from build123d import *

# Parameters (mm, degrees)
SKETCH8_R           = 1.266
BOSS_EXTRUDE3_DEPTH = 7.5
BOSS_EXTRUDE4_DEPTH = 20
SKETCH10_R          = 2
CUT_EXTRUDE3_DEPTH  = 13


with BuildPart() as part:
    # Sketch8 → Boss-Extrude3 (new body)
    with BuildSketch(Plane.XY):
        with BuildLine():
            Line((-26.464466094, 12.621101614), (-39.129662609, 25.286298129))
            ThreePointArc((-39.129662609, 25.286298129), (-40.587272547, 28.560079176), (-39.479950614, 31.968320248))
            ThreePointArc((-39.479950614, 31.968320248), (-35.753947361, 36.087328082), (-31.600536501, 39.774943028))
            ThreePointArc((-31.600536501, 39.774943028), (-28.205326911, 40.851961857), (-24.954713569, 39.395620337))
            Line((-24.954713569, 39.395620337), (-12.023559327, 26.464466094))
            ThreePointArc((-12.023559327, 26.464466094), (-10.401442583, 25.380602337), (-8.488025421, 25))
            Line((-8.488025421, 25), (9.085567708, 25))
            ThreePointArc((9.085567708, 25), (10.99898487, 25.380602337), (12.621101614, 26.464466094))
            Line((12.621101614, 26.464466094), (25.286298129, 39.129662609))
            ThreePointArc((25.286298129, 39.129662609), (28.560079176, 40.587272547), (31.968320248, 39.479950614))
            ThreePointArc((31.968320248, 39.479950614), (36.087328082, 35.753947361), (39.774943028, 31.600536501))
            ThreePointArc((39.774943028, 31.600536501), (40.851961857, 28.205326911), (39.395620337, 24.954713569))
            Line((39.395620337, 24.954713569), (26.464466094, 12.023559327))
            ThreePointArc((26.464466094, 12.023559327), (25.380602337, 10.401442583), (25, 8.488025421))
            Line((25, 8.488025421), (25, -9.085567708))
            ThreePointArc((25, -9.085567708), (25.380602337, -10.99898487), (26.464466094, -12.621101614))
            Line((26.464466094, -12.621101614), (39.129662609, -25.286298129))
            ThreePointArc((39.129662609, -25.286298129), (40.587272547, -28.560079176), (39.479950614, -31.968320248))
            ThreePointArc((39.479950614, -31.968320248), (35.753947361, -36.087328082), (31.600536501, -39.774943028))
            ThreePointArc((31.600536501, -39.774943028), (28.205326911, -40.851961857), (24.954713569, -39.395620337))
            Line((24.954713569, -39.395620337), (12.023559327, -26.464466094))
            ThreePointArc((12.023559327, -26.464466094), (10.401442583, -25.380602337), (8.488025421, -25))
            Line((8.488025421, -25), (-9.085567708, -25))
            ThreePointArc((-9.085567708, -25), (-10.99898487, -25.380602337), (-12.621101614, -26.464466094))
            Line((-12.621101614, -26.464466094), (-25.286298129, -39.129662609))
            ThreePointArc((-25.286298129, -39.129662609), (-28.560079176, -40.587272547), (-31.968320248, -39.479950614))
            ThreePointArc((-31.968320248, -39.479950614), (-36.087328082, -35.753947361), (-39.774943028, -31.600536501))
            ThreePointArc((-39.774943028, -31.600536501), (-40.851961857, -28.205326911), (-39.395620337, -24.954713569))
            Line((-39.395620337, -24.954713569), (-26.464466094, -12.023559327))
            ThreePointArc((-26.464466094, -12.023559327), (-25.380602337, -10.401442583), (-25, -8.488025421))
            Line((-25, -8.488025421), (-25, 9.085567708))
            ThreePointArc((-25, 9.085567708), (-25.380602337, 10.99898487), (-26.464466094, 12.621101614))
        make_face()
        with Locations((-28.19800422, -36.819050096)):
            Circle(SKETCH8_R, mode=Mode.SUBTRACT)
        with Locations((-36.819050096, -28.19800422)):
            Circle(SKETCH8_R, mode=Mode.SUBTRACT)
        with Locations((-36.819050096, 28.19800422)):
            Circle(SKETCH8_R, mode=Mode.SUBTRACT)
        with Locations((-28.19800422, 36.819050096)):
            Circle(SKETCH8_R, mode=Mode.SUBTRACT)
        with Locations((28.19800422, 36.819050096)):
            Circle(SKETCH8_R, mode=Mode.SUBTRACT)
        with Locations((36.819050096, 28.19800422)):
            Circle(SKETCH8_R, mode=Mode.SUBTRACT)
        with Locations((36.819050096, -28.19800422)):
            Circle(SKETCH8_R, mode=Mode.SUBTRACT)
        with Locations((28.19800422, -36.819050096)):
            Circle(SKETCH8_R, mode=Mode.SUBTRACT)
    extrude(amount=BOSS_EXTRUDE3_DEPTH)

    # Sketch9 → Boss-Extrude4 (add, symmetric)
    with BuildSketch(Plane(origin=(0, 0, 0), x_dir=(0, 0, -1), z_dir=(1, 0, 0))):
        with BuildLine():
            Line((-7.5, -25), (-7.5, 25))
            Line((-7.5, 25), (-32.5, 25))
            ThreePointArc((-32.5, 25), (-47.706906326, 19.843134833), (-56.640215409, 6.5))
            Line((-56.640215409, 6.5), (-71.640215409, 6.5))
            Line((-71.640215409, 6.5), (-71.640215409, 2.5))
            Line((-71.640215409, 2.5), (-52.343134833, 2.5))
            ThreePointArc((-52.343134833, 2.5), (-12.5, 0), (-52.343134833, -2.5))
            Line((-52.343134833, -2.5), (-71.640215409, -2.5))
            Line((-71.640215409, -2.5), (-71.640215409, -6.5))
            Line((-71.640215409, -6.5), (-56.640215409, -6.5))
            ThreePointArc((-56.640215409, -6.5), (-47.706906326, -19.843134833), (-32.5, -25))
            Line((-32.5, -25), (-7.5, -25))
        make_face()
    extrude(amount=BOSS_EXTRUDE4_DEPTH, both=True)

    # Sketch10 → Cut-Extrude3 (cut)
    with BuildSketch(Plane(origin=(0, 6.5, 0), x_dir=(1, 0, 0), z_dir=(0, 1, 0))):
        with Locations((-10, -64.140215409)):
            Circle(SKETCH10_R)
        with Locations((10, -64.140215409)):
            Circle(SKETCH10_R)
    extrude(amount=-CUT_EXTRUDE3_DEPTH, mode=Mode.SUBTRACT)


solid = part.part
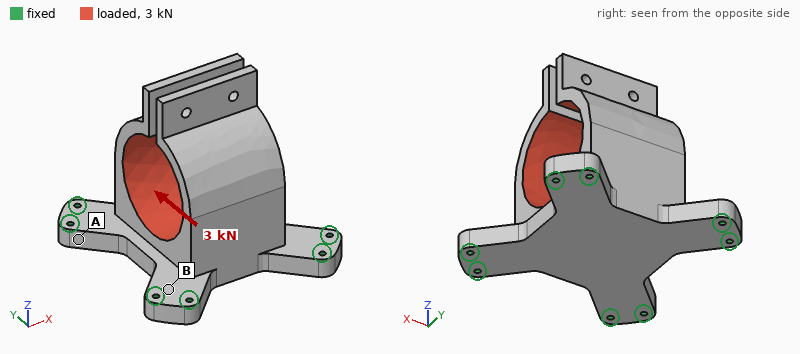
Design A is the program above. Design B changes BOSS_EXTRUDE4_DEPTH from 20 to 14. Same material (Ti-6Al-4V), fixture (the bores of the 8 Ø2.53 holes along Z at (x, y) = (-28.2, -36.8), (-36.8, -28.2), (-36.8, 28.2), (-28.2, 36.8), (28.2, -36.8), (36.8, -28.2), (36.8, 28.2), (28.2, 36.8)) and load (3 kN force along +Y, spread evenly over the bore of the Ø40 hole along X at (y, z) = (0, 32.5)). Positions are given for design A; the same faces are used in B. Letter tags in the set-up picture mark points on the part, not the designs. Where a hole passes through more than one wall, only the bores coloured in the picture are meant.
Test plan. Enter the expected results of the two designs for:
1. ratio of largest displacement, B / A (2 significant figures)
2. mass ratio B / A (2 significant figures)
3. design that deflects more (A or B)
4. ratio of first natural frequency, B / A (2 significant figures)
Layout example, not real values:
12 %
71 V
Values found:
1.5
0.82
B
1.0
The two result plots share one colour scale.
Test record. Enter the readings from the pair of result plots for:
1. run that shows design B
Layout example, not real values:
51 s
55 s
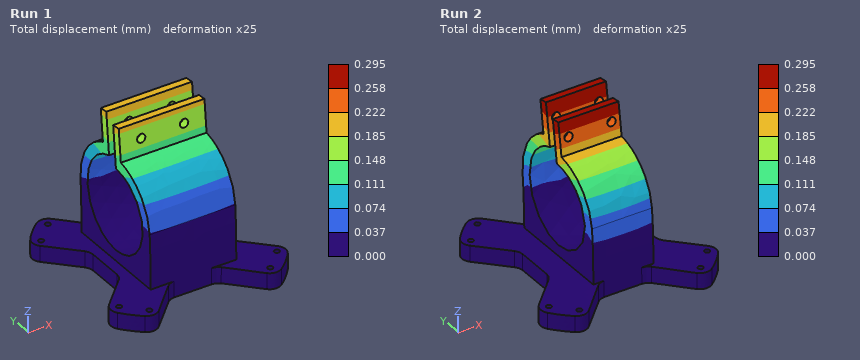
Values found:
Run 2
